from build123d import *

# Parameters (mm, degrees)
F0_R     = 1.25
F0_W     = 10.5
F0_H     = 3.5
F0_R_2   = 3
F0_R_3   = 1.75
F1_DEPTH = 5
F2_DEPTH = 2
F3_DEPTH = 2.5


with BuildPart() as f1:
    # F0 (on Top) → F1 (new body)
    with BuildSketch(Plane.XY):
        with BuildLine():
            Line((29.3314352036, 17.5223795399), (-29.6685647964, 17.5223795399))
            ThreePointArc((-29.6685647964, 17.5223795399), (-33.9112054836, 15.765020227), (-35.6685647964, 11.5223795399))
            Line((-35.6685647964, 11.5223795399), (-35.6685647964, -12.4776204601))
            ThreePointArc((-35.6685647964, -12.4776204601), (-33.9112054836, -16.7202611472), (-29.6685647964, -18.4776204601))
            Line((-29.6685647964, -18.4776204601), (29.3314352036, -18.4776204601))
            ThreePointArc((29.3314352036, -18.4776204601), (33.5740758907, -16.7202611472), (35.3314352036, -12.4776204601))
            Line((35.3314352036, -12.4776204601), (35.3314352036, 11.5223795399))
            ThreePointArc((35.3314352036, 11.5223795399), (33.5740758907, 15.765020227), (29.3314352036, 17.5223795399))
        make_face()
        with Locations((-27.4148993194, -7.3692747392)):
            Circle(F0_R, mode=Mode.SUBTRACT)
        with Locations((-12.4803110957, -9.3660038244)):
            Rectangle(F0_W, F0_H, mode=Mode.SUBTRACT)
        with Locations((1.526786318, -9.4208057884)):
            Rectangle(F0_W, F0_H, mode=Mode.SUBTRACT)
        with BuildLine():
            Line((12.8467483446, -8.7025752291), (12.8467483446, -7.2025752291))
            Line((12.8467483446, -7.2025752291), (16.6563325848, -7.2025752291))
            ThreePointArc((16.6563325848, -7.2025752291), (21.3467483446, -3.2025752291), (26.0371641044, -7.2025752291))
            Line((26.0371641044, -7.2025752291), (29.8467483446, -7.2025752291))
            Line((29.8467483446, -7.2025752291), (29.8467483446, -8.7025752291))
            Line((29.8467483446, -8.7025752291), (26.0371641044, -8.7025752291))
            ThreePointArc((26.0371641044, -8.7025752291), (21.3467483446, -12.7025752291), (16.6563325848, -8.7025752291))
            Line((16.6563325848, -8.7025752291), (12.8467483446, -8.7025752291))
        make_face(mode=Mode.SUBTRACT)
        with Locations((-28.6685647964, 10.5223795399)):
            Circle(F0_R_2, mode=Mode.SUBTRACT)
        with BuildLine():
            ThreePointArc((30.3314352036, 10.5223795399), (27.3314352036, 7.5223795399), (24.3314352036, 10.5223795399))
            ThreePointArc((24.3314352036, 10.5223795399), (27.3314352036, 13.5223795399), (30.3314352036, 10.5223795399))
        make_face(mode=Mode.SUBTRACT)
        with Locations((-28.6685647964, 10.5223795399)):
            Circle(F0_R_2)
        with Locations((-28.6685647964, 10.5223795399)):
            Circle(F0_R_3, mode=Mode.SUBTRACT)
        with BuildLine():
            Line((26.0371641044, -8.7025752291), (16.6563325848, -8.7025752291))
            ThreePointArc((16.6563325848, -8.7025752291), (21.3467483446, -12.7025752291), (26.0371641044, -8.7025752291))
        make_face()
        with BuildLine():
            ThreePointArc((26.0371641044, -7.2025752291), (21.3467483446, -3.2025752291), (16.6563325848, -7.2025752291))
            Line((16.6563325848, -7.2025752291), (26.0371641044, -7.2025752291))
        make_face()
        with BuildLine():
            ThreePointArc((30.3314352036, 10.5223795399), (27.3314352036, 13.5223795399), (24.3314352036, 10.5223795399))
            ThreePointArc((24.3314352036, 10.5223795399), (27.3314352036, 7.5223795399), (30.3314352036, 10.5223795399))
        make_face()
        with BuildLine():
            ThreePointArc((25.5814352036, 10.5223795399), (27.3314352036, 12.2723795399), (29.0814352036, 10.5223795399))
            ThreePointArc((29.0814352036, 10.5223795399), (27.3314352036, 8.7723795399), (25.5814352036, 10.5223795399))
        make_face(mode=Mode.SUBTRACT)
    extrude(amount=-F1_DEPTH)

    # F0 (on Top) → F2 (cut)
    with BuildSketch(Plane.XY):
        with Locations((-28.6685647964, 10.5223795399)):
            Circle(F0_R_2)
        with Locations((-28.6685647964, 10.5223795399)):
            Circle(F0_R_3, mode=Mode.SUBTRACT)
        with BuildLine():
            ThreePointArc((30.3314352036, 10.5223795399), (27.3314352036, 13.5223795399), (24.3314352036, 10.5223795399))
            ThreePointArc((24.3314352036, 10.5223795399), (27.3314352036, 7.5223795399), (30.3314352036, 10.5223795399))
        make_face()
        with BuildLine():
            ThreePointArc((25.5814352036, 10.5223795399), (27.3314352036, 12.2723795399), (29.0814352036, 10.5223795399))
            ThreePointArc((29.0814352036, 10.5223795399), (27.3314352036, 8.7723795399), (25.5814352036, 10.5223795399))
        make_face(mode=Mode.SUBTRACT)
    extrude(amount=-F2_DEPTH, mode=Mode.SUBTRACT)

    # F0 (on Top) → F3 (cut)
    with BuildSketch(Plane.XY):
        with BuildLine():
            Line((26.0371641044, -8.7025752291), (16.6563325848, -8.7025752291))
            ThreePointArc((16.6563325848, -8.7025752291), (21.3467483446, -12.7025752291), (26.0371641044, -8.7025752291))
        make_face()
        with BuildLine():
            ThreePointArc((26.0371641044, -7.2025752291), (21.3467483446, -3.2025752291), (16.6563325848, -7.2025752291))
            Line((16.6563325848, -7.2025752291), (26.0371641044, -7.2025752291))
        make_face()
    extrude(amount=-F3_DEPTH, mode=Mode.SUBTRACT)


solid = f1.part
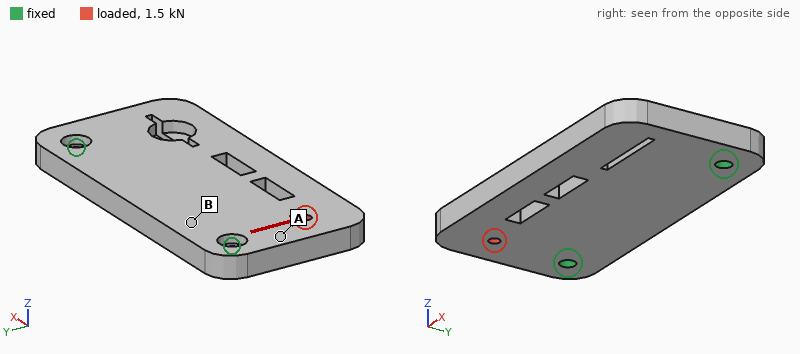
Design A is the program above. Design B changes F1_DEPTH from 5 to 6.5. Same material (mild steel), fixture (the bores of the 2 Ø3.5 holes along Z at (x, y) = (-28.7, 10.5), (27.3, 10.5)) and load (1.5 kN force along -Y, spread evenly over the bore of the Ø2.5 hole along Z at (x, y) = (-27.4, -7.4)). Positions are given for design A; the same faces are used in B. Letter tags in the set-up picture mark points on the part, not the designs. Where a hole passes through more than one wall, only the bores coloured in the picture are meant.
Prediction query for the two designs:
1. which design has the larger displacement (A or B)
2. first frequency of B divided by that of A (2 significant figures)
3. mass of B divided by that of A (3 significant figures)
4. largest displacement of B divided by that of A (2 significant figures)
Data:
A
1.3
1.31
0.48
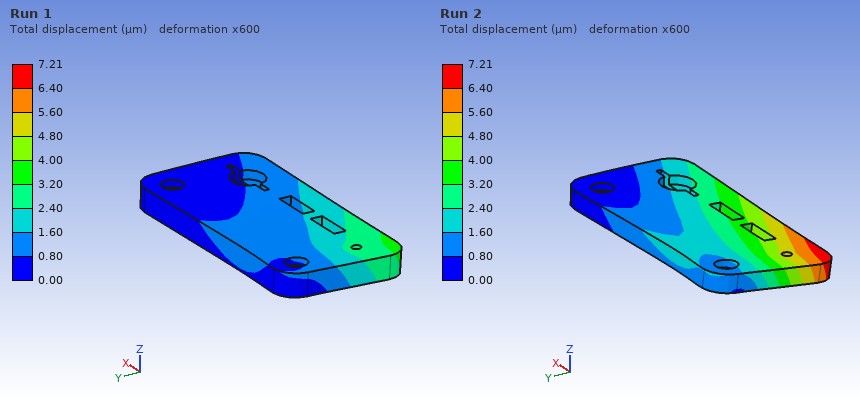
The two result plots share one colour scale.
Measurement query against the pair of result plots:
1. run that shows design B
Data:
Run 1
